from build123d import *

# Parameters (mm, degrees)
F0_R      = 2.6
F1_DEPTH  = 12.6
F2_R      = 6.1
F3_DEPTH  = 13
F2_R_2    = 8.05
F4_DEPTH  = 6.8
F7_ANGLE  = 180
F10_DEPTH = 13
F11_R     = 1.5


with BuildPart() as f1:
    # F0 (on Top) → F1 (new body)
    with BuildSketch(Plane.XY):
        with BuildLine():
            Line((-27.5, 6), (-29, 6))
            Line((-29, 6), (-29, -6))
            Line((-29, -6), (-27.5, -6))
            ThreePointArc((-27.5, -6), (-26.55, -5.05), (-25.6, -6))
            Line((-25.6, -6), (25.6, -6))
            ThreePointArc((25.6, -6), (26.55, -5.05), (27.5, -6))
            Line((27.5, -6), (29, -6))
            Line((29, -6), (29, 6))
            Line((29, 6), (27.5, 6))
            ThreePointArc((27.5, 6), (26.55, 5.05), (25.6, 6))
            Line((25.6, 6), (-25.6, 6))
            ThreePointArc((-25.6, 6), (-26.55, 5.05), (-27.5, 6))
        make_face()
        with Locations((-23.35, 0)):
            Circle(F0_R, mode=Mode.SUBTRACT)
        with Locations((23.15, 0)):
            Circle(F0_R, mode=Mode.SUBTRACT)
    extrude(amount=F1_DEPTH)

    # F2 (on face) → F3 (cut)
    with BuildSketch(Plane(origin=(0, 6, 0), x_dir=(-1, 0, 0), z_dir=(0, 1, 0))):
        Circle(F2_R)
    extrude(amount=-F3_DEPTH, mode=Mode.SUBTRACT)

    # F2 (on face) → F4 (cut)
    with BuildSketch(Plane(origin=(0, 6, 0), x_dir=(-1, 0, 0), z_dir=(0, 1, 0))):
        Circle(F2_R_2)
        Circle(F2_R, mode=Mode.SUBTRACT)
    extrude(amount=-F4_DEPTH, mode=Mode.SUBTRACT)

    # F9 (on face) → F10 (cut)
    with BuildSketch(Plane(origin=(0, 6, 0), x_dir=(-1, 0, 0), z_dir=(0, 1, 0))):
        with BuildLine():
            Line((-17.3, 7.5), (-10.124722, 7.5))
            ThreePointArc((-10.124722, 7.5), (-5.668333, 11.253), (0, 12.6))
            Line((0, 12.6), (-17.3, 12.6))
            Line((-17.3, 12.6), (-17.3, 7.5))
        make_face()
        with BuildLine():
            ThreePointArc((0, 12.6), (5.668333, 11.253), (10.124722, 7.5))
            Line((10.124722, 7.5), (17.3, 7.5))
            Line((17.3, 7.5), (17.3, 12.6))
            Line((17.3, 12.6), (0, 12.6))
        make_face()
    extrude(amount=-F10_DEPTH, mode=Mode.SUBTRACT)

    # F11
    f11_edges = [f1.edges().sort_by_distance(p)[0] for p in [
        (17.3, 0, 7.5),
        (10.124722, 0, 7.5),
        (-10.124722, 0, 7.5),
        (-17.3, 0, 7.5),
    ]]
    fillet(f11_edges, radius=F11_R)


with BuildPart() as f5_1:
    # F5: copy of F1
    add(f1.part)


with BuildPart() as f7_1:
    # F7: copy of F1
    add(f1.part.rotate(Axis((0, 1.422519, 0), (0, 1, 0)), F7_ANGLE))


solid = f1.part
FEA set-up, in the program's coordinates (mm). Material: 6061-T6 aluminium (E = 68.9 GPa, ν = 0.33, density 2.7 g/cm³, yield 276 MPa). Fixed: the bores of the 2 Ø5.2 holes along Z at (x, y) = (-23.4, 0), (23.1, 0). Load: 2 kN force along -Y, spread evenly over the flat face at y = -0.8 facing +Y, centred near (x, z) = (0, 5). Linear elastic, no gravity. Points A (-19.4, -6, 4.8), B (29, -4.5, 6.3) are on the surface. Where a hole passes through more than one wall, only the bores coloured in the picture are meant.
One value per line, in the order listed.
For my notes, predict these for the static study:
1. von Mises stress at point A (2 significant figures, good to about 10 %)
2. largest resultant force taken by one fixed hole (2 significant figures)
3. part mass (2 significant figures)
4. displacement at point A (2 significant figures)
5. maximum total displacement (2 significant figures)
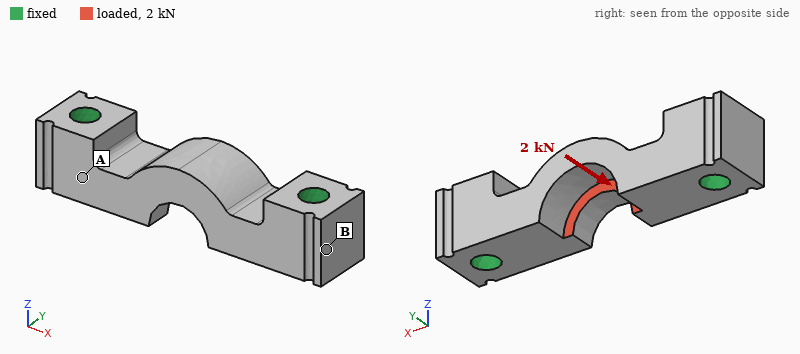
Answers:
43 MPa
1.0 kN
16 g
5.1 µm
31 µm
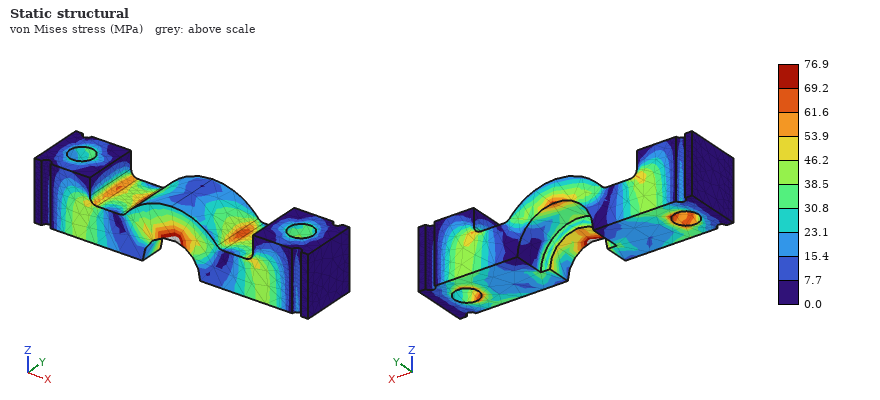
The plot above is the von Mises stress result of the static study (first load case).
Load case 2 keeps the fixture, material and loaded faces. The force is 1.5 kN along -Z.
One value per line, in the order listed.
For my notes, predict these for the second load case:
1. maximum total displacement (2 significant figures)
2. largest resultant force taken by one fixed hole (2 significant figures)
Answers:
20 µm
1.0 kN
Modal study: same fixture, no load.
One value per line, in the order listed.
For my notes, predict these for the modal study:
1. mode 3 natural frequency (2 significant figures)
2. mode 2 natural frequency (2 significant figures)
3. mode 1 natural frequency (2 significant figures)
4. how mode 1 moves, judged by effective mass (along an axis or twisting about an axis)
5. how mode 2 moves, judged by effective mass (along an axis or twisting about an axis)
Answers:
35 kHz
22 kHz
18 kHz
along Y
along Z
